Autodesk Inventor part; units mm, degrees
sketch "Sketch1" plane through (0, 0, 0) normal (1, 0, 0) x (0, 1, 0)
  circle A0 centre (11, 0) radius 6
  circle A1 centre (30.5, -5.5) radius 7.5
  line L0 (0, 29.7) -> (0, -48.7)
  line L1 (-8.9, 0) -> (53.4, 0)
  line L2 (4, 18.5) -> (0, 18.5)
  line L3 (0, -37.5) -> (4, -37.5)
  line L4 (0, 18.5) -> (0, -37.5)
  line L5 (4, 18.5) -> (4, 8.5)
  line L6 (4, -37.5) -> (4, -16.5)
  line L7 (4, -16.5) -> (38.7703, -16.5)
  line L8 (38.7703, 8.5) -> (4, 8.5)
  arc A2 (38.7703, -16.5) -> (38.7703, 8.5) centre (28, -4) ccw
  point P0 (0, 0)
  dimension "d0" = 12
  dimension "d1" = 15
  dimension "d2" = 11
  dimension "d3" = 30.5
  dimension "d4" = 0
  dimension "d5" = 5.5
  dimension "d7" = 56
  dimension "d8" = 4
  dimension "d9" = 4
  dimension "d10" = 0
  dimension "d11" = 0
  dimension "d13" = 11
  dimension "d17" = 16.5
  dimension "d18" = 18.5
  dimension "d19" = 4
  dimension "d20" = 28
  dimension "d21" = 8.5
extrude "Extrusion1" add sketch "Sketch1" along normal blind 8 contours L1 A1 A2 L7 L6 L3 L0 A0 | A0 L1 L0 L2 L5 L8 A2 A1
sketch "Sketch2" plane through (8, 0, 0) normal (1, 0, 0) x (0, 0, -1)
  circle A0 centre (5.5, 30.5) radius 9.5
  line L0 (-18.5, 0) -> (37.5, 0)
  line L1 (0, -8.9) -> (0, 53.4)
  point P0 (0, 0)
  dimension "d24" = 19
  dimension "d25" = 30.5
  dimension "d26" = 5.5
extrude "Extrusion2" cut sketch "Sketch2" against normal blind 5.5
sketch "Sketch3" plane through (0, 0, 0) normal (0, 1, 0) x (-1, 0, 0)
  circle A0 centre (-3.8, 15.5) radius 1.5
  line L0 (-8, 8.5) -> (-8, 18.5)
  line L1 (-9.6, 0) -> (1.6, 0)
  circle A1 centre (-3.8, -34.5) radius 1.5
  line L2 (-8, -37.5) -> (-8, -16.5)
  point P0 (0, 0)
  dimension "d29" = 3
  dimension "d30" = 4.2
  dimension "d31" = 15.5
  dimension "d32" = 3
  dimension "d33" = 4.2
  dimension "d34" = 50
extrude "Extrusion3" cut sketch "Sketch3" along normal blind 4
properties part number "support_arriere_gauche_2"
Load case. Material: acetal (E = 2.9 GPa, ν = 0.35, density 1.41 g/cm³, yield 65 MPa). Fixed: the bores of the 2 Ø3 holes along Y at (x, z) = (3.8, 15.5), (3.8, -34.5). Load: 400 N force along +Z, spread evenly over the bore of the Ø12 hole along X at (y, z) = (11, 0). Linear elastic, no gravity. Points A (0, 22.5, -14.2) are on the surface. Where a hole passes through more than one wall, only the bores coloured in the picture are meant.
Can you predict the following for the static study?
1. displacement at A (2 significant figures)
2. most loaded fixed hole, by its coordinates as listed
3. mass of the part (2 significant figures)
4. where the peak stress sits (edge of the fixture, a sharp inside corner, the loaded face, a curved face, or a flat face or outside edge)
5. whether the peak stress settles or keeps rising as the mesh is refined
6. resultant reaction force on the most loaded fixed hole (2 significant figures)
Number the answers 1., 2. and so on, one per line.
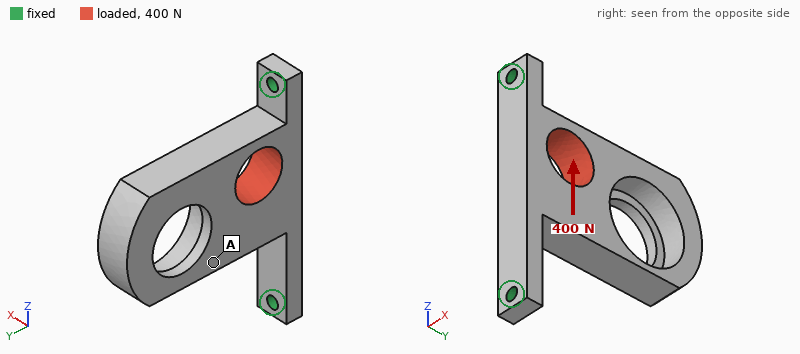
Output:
1. 0.52 mm
2. (3.8, 15.5)
3. 9.3 g
4. edge of the fixture
5. keeps rising
6. 260 N
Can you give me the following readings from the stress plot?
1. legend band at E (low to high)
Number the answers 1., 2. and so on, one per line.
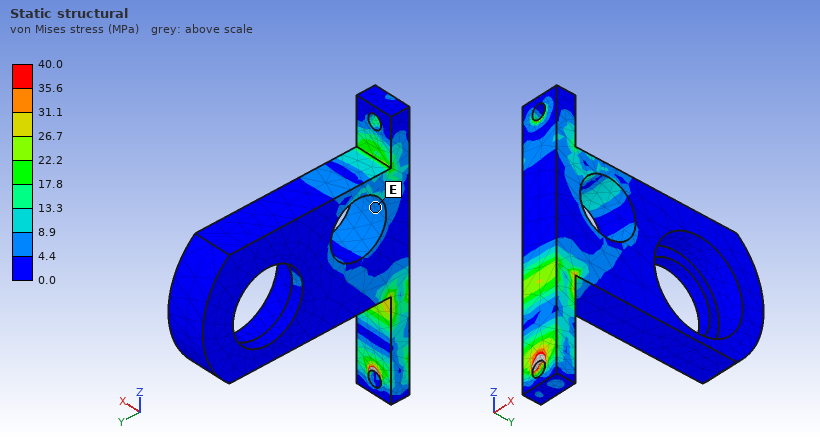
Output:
1. 4.4 to 8.9 MPa
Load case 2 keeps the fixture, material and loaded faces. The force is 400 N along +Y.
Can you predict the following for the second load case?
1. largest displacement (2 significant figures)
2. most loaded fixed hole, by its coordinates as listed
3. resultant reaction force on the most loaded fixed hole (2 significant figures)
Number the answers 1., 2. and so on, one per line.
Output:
1. 0.72 mm
2. (3.8, 15.5)
3. 300 N
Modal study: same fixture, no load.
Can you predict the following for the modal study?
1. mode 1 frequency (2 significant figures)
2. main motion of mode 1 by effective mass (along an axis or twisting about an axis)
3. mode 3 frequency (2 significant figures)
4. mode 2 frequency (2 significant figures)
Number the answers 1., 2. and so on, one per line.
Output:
1. 360 Hz
2. along X
3. 2000 Hz
4. 930 Hz
